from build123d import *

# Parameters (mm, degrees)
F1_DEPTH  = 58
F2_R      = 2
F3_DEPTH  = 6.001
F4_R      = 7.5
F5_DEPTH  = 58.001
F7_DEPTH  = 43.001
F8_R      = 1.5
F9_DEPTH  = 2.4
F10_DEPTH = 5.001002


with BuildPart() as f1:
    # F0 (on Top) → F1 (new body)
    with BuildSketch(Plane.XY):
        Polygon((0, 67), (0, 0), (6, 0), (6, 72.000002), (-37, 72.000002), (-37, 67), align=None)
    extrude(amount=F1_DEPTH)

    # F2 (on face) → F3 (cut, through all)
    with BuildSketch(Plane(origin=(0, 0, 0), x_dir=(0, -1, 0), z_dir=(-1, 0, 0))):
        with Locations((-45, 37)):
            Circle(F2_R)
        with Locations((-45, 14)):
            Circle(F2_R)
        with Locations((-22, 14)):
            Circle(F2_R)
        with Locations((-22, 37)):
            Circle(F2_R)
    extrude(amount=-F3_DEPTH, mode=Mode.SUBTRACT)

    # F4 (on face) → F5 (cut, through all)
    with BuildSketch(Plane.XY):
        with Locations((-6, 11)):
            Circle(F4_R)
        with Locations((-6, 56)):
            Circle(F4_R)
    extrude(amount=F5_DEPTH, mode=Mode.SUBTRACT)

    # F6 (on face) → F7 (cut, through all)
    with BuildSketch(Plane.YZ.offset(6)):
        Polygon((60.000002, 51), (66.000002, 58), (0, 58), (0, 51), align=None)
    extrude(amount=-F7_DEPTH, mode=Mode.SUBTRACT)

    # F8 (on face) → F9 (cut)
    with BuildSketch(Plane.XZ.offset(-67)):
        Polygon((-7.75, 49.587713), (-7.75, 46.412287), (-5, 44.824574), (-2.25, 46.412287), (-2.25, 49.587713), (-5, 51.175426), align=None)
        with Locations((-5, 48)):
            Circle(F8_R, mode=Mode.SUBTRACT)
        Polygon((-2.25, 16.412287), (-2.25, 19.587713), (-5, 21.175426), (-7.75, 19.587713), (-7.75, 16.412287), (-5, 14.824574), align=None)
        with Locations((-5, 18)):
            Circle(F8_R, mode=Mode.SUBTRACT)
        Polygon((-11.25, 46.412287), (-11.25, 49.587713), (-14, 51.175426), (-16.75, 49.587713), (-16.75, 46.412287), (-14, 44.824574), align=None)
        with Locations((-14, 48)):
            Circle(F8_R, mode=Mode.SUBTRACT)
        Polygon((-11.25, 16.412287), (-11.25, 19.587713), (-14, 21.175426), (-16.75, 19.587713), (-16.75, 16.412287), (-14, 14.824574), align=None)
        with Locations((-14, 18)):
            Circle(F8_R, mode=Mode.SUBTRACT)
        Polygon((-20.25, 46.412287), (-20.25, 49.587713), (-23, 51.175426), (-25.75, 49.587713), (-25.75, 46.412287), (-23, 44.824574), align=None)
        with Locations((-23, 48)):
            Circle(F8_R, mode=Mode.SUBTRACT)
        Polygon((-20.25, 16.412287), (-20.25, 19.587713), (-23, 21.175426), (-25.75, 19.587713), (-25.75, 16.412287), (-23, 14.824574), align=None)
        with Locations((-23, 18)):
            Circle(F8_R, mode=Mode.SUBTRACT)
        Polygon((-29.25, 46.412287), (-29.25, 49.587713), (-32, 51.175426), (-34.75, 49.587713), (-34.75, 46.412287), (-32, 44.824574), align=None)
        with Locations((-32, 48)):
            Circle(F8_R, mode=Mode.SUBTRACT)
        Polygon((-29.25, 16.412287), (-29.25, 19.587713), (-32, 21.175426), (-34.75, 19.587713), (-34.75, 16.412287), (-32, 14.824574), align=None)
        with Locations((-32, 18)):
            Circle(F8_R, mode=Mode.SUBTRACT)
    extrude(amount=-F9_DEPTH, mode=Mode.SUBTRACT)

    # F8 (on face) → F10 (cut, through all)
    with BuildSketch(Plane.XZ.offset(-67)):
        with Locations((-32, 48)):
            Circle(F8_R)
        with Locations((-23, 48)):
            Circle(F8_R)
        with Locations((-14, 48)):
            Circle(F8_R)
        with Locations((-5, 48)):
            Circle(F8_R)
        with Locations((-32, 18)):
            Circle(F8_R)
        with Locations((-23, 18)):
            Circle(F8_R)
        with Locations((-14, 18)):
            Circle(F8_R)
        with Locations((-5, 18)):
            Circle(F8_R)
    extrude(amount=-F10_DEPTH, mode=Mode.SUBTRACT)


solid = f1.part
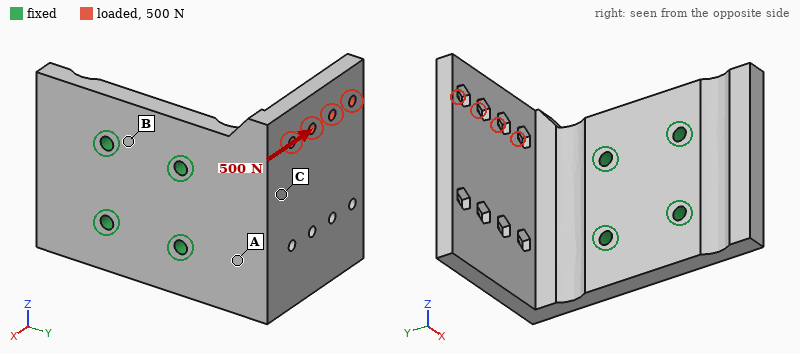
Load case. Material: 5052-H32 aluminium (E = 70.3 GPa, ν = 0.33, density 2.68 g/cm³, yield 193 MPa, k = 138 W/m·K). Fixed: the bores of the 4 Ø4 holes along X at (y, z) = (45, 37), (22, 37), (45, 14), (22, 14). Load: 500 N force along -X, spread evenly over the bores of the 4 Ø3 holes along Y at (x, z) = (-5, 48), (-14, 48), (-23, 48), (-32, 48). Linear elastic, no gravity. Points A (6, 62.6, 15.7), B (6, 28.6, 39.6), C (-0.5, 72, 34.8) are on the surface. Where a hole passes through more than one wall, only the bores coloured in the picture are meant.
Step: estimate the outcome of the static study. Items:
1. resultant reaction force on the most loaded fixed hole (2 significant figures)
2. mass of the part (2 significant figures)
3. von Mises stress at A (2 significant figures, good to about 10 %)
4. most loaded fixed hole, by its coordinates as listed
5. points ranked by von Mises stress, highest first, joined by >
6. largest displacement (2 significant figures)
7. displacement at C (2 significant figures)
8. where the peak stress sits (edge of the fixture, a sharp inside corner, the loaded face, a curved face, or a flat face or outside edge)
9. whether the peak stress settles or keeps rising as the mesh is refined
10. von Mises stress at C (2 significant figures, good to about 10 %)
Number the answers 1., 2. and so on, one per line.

1. 760 N
2. 84 g
3. 25 MPa
4. (45, 37)
5. A > C > B
6. 0.24 mm
7. 0.085 mm
8. edge of the fixture
9. keeps rising
10. 15 MPa
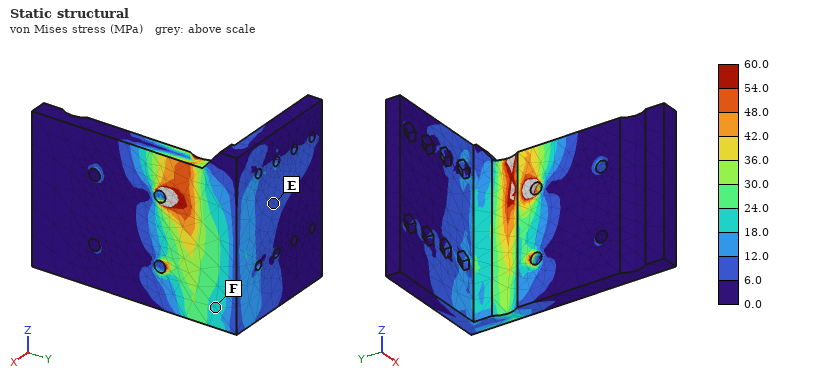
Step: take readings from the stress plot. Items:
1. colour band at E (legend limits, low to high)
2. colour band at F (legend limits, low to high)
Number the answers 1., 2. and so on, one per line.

1. 6.0 to 12.0 MPa
2. 18.0 to 24.0 MPa
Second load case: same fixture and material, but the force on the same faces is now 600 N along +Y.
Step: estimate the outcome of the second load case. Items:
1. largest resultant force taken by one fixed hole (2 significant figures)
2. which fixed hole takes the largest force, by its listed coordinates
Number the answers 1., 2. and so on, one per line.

1. 570 N
2. (45, 37)
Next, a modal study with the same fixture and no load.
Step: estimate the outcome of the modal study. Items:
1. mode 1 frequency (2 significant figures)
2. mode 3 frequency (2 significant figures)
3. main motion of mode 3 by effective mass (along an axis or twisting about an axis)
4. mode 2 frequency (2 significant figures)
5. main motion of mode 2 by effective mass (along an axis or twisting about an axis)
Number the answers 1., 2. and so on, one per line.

1. 1400 Hz
2. 4100 Hz
3. along X
4. 2400 Hz
5. along Z
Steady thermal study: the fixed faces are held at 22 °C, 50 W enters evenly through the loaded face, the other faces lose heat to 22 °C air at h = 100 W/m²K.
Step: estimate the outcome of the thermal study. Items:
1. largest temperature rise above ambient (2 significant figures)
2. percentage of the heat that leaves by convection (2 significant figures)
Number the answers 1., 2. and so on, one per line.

1. 61 K
2. 44 %
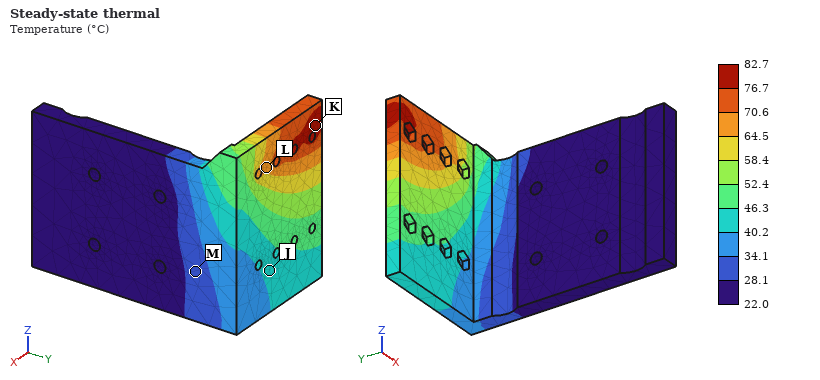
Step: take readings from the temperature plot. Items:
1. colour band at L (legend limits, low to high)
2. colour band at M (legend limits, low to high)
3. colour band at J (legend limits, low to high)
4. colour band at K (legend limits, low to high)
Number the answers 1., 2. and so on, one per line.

1. 64.5 to 70.6 °C
2. 28.1 to 34.1 °C
3. 40.2 to 46.3 °C
4. 76.7 to 82.7 °C
